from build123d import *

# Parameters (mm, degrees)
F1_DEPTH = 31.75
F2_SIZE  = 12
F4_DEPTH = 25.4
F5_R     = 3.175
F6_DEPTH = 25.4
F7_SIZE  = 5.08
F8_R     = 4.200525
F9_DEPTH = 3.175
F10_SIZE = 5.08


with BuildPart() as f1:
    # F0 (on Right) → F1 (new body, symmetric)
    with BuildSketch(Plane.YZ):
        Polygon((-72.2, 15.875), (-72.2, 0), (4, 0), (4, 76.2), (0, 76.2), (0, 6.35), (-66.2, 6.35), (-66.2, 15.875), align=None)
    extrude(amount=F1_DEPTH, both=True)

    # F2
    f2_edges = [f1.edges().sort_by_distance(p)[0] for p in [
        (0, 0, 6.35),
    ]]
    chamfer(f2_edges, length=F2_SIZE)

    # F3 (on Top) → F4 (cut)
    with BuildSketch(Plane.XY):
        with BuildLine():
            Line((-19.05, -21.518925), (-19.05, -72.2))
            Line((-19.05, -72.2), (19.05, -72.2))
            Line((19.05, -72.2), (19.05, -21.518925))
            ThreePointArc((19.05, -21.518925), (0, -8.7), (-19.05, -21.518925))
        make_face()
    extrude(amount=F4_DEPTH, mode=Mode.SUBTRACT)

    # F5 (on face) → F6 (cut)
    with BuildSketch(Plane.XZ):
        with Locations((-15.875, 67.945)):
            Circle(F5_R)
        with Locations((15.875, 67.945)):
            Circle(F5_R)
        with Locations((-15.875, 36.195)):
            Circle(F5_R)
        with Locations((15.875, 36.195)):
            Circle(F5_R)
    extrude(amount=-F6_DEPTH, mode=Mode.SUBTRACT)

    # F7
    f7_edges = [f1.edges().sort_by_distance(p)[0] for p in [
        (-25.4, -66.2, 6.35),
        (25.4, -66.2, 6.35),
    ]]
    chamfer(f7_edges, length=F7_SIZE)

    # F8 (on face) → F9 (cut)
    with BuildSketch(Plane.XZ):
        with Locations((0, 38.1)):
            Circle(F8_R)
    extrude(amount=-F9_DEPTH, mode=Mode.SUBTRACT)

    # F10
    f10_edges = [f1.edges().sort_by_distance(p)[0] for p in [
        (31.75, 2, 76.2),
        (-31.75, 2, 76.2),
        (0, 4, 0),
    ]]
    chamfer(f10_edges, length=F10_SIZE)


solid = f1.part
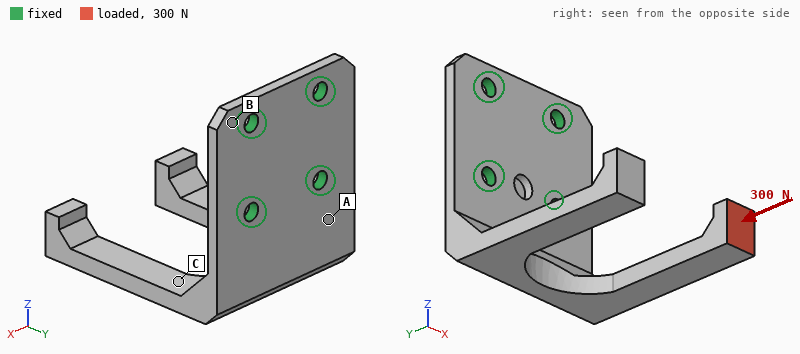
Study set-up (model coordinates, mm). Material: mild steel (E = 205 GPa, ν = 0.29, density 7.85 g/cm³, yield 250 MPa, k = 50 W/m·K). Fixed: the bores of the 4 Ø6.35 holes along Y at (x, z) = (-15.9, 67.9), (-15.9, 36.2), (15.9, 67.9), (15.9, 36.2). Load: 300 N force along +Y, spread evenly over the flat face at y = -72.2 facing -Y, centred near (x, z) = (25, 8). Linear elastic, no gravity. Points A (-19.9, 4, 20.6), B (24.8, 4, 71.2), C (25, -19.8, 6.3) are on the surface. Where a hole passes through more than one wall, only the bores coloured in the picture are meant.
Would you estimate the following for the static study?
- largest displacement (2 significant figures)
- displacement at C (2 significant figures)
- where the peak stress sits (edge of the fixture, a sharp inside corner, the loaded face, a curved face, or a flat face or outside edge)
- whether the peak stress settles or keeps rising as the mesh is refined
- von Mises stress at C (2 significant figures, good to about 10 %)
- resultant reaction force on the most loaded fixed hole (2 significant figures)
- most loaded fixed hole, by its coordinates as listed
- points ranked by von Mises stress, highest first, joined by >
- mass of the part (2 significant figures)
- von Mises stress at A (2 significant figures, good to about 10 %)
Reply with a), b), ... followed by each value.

a) 0.11 mm
b) 0.055 mm
c) edge of the fixture
d) keeps rising
e) 19 MPa
f) 370 N
g) (15.9, 36.2)
h) A > C > B
i) 300 g
j) 28 MPa
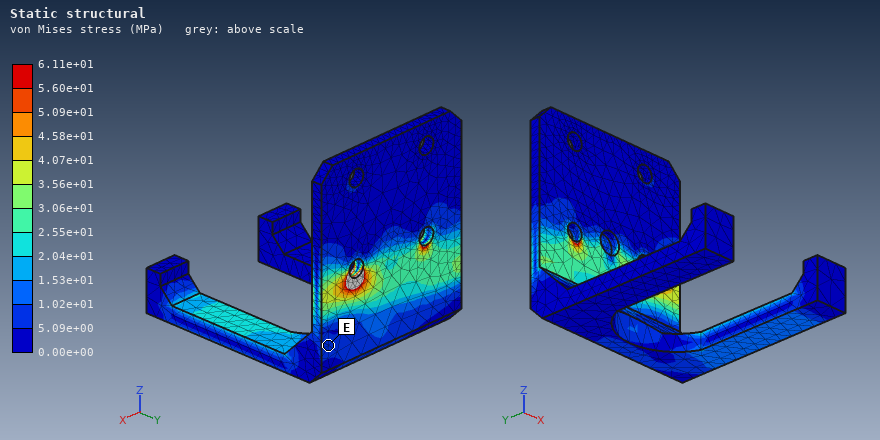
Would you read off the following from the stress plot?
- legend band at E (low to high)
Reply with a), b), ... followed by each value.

a) 5.09e+00 to 1.02e+01 MPa
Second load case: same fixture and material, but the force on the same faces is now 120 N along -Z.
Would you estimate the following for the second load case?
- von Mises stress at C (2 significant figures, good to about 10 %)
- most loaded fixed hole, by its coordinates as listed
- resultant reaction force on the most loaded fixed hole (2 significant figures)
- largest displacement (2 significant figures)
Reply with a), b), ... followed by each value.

a) 68 MPa
b) (15.9, 36.2)
c) 130 N
d) 0.38 mm
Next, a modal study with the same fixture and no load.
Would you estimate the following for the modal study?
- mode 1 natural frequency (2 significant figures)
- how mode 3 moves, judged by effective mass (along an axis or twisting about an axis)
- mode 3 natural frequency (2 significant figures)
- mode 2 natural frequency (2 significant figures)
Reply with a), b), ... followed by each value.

a) 490 Hz
b) along X
c) 1200 Hz
d) 930 Hz
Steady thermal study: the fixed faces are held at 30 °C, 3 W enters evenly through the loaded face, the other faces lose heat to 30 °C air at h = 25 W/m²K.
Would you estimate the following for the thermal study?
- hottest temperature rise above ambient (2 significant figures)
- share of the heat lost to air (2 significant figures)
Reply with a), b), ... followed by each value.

a) 35 K
b) 58 %
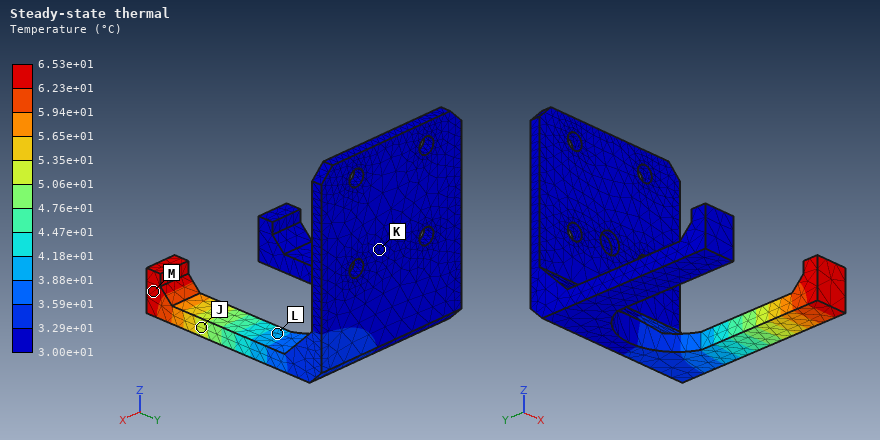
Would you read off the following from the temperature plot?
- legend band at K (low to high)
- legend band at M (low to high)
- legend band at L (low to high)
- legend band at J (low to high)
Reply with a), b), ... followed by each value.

a) 3.00e+01 to 3.29e+01 °C
b) 6.23e+01 to 6.53e+01 °C
c) 3.88e+01 to 4.18e+01 °C
d) 5.06e+01 to 5.35e+01 °C
